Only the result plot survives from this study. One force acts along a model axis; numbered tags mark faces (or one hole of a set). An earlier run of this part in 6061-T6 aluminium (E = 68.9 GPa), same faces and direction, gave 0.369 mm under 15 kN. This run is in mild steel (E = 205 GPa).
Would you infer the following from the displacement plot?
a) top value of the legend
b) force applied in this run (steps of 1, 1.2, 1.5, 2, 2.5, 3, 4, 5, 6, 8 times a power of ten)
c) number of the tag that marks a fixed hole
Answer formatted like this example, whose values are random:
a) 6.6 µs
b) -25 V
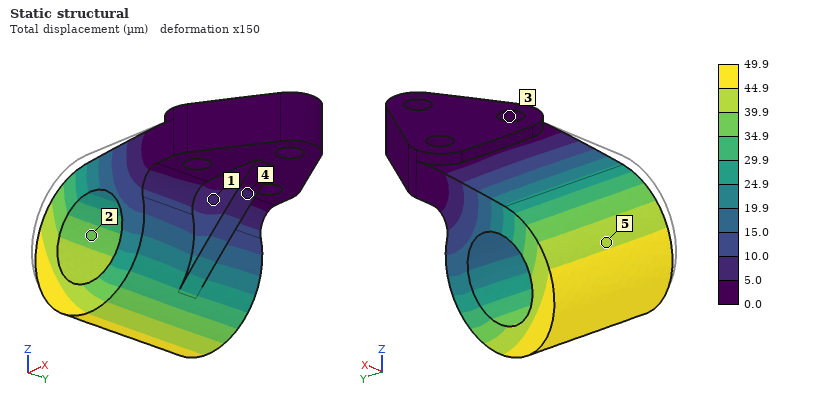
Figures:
a) 49.9 µm
b) 6 kN
c) 3
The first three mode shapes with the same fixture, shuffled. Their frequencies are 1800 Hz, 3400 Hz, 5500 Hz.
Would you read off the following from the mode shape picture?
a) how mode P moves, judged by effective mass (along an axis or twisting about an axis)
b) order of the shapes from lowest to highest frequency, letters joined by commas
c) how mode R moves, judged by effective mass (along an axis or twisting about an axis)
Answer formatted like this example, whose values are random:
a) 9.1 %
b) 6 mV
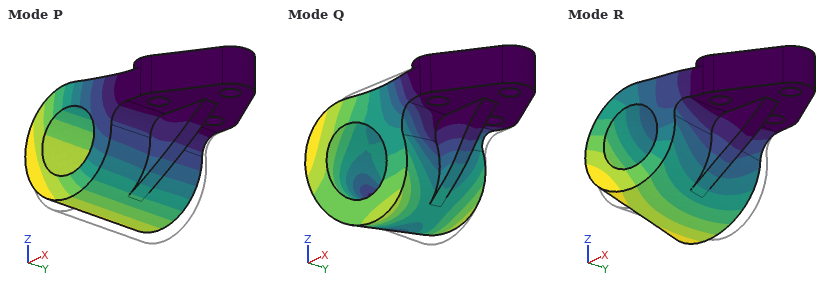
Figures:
a) along Z
b) P, R, Q
c) along Y
